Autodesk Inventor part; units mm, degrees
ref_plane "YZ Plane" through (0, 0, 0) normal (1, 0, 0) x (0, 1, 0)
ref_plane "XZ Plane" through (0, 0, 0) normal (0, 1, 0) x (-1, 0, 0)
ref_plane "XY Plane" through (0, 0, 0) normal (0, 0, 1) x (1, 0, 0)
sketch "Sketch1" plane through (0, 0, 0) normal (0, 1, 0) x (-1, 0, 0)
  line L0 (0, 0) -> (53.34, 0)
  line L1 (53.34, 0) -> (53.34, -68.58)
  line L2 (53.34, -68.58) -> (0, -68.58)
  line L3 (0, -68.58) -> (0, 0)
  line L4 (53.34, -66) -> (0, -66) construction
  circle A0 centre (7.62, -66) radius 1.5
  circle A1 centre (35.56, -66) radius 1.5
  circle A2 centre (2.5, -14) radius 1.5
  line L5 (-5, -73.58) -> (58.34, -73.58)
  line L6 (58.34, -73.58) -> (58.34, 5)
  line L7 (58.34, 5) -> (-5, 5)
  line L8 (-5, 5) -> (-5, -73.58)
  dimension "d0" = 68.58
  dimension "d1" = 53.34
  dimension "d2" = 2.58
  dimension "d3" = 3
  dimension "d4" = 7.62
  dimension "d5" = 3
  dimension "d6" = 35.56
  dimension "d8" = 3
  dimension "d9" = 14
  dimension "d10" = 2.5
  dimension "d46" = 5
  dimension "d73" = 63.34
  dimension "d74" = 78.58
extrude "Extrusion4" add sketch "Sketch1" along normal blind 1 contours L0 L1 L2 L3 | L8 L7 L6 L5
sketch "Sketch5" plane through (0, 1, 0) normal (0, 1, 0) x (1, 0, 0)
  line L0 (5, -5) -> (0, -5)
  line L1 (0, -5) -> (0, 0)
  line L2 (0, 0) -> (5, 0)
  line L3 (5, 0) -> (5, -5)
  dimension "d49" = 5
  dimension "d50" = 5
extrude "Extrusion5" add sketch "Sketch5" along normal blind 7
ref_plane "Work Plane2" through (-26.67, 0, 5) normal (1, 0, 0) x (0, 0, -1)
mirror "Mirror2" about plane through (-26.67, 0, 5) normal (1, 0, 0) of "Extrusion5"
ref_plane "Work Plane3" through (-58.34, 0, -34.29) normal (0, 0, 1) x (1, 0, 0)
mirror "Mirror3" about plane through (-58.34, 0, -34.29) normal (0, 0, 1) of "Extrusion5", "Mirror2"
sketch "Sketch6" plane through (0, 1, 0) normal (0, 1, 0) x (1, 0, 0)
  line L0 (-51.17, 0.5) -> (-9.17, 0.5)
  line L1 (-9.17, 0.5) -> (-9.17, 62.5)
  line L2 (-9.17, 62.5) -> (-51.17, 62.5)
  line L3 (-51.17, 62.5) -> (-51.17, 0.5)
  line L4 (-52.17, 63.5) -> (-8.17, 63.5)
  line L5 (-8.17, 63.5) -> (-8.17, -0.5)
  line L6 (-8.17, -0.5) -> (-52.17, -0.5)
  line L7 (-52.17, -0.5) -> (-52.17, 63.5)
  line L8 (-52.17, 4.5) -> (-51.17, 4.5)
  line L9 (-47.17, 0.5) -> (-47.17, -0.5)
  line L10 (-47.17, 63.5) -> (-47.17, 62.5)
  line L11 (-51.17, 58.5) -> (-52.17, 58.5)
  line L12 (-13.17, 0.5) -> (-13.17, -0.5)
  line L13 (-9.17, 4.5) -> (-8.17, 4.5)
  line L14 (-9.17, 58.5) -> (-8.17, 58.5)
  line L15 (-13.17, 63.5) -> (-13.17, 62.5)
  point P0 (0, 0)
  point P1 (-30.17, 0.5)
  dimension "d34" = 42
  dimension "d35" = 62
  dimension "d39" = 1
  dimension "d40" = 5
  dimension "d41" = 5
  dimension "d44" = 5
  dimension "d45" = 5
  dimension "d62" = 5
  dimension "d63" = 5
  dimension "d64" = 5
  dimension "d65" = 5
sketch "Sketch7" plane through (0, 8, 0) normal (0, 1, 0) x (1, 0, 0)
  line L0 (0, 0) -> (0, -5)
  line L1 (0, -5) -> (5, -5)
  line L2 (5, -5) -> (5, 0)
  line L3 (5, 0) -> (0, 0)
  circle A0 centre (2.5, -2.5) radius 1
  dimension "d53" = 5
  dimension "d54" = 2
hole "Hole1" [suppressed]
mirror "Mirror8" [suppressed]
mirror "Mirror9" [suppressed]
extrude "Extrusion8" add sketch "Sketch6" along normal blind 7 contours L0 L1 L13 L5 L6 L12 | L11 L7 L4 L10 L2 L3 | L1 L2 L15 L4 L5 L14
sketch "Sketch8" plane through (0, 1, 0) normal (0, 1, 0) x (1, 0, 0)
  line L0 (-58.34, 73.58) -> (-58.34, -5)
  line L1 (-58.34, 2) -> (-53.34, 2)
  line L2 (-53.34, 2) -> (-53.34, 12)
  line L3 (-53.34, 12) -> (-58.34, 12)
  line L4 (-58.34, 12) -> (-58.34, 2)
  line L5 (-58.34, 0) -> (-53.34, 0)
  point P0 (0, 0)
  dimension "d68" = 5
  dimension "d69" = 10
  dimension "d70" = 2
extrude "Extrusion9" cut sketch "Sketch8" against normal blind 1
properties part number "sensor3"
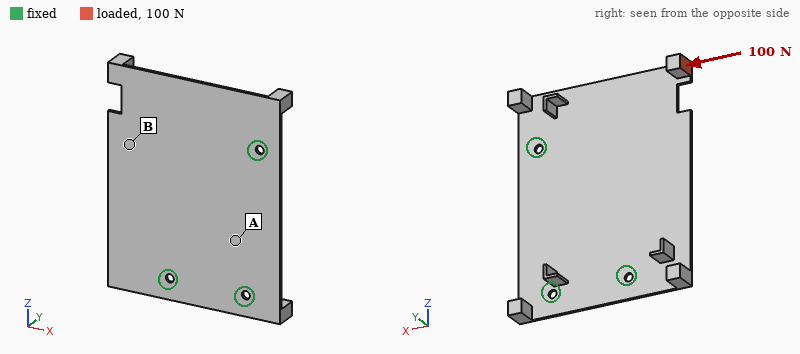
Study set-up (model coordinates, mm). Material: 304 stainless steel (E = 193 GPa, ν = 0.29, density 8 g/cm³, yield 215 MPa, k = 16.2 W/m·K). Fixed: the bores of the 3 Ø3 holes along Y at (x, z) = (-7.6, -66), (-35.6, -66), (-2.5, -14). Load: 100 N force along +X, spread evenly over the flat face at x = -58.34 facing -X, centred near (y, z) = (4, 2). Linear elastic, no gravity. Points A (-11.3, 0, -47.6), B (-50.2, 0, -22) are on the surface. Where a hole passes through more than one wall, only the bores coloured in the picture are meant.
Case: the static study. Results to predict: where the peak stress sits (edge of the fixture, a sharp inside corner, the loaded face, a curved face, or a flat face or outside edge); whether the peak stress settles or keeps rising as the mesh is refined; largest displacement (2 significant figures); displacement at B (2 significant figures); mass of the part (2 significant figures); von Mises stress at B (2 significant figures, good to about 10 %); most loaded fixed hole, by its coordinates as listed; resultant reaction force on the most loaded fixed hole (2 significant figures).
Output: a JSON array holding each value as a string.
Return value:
["a sharp inside corner", "keeps rising", "0.67 mm", "0.22 mm", "46 g", "39 MPa", "(-2.5, -14)", "110 N"]
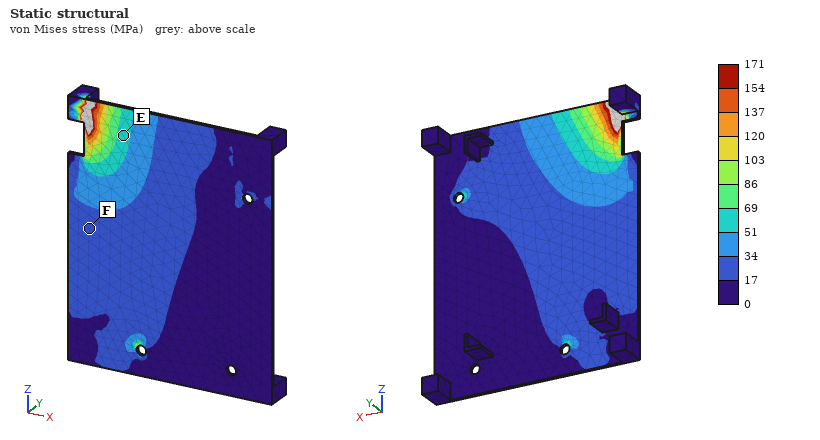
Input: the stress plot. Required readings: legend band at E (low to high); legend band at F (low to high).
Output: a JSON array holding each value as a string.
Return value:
["51 to 69 MPa", "17 to 34 MPa"]
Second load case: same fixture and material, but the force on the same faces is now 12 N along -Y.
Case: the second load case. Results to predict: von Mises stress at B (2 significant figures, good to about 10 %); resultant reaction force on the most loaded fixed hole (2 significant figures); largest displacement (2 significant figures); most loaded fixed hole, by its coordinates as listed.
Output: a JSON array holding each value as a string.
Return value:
["40 MPa", "11 N", "0.89 mm", "(-2.5, -14)"]
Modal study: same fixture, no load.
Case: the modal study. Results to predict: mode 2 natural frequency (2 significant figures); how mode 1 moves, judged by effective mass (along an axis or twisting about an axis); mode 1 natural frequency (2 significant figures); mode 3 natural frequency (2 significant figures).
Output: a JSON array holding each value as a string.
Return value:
["880 Hz", "along Y", "320 Hz", "1200 Hz"]
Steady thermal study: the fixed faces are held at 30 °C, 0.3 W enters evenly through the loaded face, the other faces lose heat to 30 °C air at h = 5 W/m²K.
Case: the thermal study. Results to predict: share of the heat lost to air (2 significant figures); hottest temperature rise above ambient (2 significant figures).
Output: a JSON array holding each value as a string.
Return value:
["59 %", "33 K"]
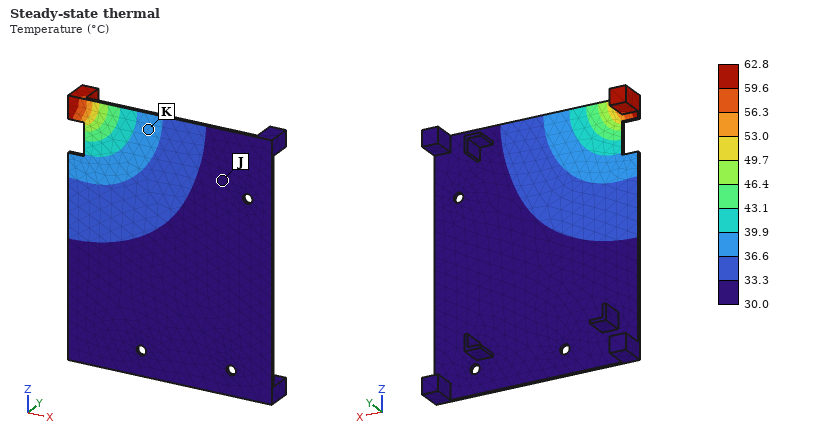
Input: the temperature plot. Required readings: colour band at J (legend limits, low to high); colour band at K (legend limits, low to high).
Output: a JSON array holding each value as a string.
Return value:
["30.0 to 33.3 °C", "36.6 to 39.9 °C"]
